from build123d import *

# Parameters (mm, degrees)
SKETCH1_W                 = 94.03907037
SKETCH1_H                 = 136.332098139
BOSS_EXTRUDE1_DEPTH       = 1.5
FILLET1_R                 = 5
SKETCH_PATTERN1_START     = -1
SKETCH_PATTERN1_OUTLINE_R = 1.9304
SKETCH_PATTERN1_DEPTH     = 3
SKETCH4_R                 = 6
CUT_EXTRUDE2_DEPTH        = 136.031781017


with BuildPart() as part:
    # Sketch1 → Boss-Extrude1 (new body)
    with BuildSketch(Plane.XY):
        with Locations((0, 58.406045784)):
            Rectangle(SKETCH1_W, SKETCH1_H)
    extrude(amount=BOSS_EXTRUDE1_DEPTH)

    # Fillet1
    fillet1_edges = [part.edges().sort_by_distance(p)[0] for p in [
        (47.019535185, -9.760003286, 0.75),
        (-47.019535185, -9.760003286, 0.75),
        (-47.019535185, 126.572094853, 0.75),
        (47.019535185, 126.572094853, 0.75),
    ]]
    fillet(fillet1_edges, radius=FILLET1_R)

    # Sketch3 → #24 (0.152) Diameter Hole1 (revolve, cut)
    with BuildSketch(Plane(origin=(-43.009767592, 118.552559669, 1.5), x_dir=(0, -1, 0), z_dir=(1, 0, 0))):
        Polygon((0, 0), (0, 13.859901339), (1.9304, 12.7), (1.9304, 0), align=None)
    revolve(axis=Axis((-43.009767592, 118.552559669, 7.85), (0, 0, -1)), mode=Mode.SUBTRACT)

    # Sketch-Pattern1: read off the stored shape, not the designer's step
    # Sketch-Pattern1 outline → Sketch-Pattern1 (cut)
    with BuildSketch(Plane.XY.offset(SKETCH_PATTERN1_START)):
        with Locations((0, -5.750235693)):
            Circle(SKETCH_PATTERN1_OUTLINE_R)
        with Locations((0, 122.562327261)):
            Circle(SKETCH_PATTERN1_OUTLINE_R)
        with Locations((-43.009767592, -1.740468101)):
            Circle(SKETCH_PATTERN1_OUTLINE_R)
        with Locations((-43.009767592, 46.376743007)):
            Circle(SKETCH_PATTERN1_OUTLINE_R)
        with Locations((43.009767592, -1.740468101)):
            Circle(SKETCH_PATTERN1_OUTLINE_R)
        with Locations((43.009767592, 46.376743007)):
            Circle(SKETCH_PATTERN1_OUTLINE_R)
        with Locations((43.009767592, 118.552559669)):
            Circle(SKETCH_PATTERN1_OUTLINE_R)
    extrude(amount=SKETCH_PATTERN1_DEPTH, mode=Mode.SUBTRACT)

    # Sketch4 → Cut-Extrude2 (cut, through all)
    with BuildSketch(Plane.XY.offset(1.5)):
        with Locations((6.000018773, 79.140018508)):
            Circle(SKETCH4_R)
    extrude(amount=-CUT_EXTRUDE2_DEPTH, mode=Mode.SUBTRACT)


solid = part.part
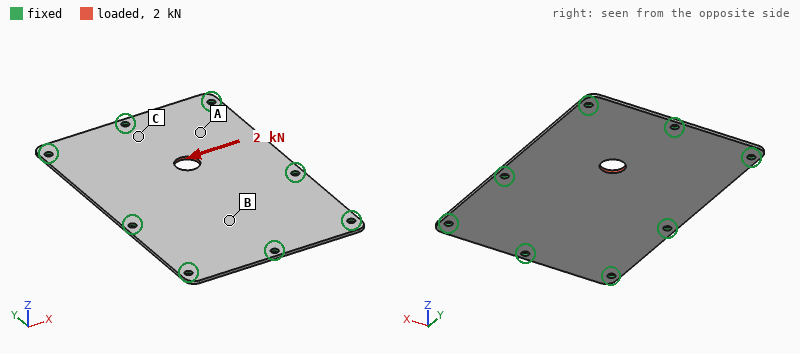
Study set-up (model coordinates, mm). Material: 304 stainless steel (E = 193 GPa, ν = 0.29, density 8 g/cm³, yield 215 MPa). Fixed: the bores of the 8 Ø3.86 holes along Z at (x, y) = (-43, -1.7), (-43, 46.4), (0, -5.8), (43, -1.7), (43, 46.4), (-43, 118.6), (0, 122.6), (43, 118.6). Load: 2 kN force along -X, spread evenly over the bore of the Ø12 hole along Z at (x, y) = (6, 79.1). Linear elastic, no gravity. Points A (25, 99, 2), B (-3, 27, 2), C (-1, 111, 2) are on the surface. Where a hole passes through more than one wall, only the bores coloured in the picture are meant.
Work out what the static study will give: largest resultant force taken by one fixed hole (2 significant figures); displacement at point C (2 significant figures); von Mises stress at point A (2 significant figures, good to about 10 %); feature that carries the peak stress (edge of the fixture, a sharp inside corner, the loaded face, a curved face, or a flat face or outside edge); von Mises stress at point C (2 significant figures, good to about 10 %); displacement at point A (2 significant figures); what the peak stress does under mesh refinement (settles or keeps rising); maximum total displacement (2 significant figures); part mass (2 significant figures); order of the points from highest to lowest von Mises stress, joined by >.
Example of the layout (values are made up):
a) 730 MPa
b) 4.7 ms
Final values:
a) 510 N
b) 1.6 µm
c) 17 MPa
d) edge of the fixture
e) 9.0 MPa
f) 2.9 µm
g) keeps rising
h) 6.2 µm
i) 150 g
j) A > C > B
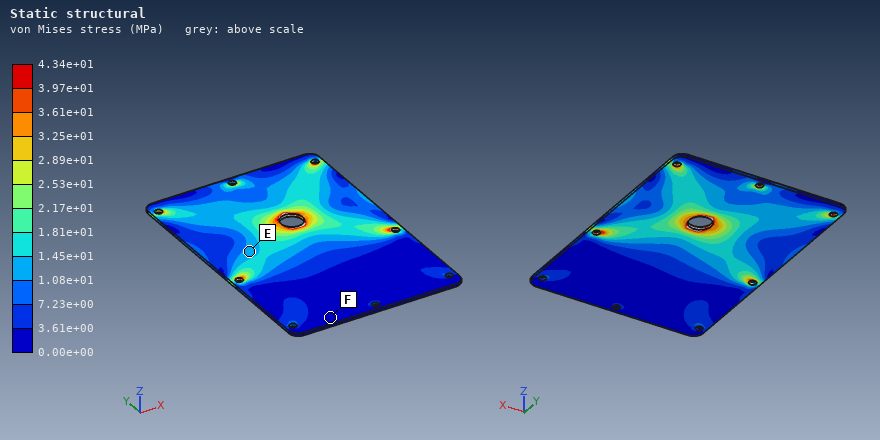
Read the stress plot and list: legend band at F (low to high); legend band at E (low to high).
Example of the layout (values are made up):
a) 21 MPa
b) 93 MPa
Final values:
a) 0.00e+00 to 3.61e+00 MPa
b) 1.08e+01 to 1.45e+01 MPa
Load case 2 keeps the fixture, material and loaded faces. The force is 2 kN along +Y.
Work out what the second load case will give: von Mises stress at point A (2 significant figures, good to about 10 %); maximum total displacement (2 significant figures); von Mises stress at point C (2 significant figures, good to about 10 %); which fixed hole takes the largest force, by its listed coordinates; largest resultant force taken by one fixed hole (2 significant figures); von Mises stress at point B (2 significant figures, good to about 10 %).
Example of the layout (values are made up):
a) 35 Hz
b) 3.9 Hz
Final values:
a) 11 MPa
b) 4.8 µm
c) 20 MPa
d) (0, 122.6)
e) 520 N
f) 6.9 MPa
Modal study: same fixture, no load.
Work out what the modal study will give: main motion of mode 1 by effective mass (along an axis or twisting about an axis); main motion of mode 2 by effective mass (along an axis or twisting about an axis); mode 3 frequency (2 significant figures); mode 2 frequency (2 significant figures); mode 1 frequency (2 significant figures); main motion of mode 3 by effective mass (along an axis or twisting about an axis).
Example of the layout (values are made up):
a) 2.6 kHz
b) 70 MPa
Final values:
a) along Z
b) twisting about X
c) 1500 Hz
d) 1500 Hz
e) 950 Hz
f) twisting about Y
